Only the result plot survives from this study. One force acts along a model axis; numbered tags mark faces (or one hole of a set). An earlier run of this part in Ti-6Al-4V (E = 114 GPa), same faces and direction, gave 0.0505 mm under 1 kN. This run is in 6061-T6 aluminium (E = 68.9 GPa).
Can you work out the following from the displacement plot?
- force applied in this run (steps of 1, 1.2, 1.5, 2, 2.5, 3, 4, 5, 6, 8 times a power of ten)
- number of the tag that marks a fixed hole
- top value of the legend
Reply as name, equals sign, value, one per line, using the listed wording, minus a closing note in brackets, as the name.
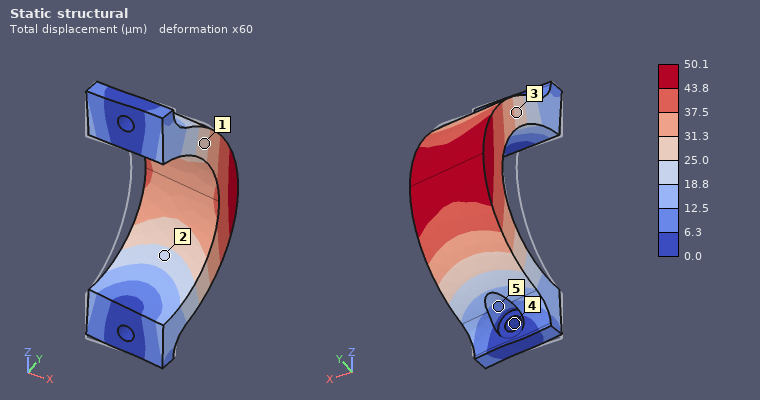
force applied in this run = 600 N
number of the tag that marks a fixed hole = 4
top value of the legend = 50.1 µm
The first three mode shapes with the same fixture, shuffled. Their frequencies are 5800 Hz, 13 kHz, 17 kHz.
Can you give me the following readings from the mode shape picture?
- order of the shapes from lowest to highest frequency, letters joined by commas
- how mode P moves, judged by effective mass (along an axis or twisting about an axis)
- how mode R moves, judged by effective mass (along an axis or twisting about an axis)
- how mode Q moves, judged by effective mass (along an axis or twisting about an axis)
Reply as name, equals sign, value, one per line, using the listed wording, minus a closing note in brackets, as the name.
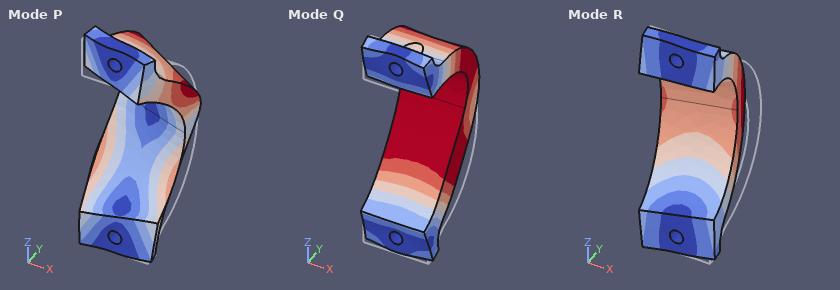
order of the shapes from lowest to highest frequency, letters joined by commas = R, Q, P
how mode P moves, judged by effective mass = twisting about Y
how mode R moves, judged by effective mass = along X
how mode Q moves, judged by effective mass = along Z
